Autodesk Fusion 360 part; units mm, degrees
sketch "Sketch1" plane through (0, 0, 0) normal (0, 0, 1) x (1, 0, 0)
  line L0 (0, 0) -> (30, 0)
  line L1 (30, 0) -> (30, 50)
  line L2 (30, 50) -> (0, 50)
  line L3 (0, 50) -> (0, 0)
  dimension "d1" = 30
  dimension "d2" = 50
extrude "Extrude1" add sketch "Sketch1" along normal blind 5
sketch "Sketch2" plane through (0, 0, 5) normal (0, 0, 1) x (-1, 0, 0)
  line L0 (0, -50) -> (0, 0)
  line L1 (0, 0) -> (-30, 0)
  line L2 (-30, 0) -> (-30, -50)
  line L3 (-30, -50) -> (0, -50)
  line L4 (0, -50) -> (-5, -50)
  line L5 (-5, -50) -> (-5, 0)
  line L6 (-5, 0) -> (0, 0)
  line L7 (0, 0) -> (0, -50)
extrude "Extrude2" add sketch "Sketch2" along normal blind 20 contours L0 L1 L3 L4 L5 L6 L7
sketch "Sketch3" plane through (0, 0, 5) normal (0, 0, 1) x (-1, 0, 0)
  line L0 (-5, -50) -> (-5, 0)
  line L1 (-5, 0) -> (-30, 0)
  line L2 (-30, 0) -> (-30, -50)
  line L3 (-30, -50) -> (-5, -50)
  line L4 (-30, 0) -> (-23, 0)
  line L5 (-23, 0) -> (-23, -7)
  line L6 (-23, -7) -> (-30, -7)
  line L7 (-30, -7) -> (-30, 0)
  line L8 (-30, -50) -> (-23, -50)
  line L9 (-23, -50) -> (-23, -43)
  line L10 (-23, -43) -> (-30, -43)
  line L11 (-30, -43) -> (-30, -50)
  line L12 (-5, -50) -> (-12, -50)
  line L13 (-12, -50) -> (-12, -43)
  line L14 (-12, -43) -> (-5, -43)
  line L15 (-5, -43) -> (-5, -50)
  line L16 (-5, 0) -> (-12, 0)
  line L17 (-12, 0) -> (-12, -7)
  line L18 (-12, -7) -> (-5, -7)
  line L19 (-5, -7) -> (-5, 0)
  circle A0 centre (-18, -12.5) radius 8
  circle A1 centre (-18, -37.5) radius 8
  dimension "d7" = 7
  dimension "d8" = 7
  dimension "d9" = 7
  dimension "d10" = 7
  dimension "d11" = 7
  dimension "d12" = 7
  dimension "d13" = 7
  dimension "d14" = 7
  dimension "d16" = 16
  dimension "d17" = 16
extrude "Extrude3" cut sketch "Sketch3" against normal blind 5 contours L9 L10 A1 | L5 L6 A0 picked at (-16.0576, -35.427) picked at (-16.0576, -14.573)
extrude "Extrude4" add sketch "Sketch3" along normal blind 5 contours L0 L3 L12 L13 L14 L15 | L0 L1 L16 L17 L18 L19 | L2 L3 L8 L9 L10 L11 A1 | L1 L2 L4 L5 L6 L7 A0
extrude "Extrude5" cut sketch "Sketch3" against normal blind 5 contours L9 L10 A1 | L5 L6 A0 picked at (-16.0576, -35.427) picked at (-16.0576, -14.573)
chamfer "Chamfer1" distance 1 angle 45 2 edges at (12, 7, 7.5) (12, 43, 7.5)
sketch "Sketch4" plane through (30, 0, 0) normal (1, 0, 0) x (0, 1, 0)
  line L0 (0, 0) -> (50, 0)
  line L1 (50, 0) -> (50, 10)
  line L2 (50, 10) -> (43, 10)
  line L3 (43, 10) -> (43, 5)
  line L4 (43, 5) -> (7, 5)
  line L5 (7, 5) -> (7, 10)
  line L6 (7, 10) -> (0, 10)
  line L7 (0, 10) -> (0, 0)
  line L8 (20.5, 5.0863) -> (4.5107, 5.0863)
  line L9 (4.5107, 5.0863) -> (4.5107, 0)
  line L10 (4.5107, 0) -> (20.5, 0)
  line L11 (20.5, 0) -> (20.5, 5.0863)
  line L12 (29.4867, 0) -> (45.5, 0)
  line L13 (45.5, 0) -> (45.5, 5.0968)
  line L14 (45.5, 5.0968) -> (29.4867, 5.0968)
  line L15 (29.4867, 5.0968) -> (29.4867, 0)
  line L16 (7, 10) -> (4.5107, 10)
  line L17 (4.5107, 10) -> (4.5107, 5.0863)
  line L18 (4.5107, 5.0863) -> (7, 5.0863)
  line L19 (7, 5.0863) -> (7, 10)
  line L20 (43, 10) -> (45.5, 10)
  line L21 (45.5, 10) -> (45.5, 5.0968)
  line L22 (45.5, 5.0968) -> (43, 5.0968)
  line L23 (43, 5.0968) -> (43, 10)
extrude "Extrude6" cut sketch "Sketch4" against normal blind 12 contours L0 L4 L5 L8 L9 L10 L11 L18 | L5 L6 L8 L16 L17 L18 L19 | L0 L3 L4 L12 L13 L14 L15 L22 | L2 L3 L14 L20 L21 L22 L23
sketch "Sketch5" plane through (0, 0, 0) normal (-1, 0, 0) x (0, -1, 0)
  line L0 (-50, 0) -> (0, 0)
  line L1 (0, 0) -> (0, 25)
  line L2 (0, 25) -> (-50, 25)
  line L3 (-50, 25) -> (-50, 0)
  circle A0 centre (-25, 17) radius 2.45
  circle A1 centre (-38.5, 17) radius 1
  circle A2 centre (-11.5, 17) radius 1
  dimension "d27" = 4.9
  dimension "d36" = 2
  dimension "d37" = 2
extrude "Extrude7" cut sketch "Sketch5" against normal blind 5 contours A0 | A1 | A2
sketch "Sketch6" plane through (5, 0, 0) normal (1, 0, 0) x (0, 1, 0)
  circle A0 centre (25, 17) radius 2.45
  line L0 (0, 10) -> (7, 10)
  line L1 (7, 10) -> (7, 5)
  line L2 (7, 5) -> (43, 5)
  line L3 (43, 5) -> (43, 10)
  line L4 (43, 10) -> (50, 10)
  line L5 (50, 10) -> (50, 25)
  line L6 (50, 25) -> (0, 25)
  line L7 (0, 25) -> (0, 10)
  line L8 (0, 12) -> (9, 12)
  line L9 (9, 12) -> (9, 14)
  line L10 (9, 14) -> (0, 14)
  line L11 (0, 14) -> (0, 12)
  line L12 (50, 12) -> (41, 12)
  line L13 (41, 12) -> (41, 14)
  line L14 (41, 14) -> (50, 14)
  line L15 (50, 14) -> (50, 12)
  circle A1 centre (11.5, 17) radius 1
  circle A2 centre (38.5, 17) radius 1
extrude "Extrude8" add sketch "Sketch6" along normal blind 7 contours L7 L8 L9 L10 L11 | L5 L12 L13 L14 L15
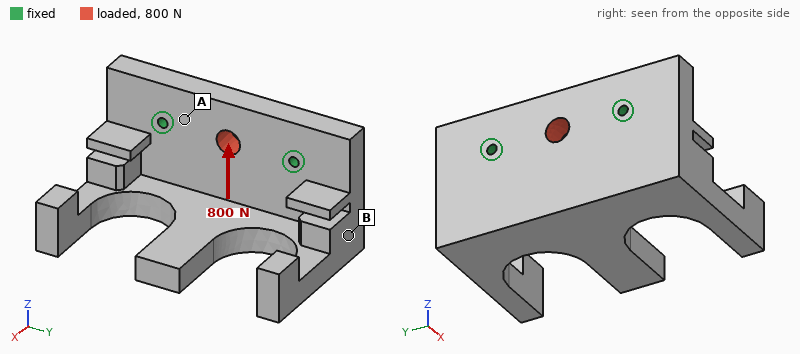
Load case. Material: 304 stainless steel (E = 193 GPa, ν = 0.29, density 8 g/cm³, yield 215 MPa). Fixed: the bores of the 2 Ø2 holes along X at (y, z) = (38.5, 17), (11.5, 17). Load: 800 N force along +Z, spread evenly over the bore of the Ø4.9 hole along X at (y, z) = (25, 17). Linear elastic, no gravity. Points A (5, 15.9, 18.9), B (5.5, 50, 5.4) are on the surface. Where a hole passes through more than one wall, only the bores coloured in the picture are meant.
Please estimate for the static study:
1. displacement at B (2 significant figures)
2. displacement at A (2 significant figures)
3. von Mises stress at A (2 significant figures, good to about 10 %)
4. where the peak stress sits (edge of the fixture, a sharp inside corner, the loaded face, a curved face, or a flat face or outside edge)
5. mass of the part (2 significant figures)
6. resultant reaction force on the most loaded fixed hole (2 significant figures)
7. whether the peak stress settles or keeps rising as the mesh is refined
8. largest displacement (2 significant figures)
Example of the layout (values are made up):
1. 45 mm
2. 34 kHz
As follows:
1. 0.27 µm
2. 0.44 µm
3. 7.2 MPa
4. edge of the fixture
5. 84 g
6. 410 N
7. keeps rising
8. 1.2 µm
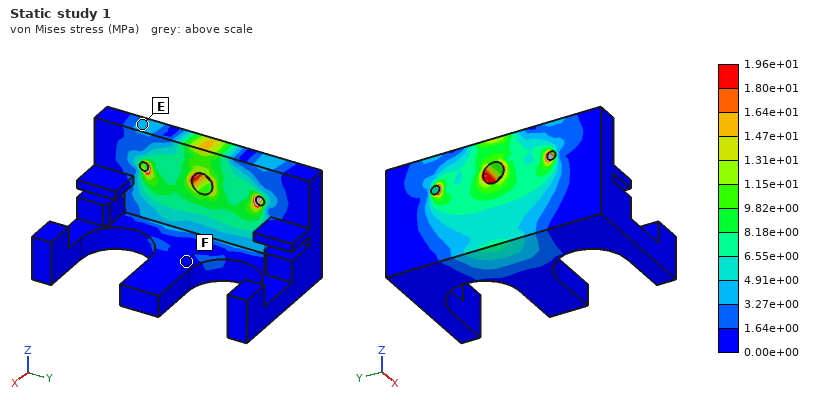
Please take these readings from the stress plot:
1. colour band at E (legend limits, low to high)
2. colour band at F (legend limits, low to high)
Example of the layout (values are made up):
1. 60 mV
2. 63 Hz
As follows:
1. 3.27e+00 to 4.91e+00 MPa
2. 0.00e+00 to 1.64e+00 MPa
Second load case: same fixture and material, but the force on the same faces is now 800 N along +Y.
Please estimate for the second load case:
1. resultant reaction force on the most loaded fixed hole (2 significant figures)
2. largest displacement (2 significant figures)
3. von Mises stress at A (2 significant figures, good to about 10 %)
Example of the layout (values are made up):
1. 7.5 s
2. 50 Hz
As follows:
1. 400 N
2. 0.59 µm
3. 8.1 MPa
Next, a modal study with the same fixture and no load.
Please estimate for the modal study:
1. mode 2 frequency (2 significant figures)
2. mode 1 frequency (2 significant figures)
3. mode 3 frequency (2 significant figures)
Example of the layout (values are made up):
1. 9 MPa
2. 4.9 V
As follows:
1. 4400 Hz
2. 3400 Hz
3. 6200 Hz
